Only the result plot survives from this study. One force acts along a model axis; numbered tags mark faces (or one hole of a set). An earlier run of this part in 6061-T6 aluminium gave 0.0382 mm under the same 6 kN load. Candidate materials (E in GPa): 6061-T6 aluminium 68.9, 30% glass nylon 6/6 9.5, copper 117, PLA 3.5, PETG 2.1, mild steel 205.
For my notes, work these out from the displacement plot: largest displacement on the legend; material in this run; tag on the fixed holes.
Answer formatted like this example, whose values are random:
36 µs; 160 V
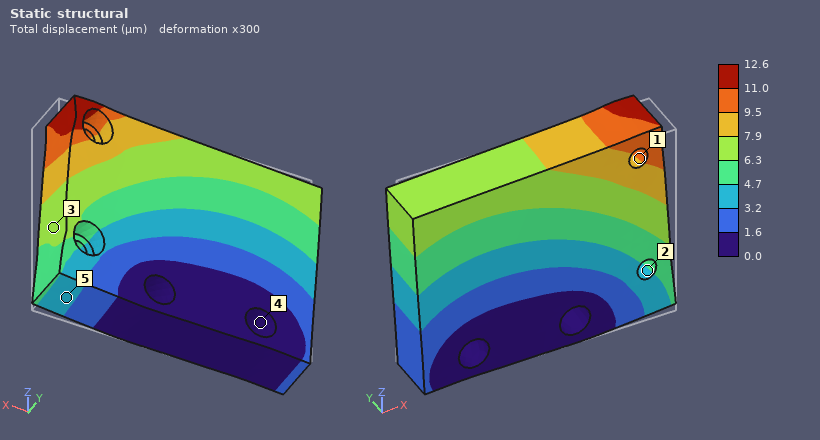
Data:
12.6 µm; mild steel; 4
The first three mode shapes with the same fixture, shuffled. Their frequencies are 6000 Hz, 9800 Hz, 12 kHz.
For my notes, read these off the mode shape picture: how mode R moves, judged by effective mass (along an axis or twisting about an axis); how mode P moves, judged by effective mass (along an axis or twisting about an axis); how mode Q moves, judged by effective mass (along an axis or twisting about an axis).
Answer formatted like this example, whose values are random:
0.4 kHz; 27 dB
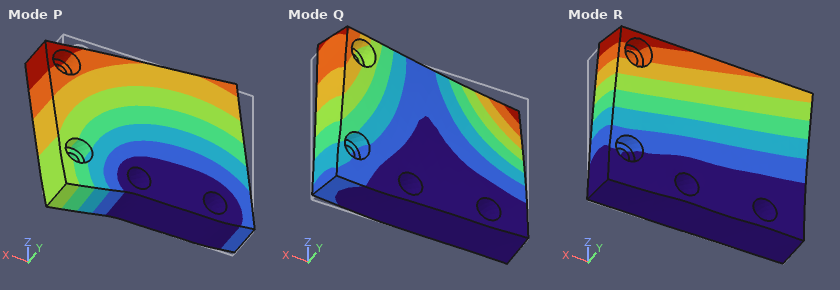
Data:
along Y; along X; twisting about Z
